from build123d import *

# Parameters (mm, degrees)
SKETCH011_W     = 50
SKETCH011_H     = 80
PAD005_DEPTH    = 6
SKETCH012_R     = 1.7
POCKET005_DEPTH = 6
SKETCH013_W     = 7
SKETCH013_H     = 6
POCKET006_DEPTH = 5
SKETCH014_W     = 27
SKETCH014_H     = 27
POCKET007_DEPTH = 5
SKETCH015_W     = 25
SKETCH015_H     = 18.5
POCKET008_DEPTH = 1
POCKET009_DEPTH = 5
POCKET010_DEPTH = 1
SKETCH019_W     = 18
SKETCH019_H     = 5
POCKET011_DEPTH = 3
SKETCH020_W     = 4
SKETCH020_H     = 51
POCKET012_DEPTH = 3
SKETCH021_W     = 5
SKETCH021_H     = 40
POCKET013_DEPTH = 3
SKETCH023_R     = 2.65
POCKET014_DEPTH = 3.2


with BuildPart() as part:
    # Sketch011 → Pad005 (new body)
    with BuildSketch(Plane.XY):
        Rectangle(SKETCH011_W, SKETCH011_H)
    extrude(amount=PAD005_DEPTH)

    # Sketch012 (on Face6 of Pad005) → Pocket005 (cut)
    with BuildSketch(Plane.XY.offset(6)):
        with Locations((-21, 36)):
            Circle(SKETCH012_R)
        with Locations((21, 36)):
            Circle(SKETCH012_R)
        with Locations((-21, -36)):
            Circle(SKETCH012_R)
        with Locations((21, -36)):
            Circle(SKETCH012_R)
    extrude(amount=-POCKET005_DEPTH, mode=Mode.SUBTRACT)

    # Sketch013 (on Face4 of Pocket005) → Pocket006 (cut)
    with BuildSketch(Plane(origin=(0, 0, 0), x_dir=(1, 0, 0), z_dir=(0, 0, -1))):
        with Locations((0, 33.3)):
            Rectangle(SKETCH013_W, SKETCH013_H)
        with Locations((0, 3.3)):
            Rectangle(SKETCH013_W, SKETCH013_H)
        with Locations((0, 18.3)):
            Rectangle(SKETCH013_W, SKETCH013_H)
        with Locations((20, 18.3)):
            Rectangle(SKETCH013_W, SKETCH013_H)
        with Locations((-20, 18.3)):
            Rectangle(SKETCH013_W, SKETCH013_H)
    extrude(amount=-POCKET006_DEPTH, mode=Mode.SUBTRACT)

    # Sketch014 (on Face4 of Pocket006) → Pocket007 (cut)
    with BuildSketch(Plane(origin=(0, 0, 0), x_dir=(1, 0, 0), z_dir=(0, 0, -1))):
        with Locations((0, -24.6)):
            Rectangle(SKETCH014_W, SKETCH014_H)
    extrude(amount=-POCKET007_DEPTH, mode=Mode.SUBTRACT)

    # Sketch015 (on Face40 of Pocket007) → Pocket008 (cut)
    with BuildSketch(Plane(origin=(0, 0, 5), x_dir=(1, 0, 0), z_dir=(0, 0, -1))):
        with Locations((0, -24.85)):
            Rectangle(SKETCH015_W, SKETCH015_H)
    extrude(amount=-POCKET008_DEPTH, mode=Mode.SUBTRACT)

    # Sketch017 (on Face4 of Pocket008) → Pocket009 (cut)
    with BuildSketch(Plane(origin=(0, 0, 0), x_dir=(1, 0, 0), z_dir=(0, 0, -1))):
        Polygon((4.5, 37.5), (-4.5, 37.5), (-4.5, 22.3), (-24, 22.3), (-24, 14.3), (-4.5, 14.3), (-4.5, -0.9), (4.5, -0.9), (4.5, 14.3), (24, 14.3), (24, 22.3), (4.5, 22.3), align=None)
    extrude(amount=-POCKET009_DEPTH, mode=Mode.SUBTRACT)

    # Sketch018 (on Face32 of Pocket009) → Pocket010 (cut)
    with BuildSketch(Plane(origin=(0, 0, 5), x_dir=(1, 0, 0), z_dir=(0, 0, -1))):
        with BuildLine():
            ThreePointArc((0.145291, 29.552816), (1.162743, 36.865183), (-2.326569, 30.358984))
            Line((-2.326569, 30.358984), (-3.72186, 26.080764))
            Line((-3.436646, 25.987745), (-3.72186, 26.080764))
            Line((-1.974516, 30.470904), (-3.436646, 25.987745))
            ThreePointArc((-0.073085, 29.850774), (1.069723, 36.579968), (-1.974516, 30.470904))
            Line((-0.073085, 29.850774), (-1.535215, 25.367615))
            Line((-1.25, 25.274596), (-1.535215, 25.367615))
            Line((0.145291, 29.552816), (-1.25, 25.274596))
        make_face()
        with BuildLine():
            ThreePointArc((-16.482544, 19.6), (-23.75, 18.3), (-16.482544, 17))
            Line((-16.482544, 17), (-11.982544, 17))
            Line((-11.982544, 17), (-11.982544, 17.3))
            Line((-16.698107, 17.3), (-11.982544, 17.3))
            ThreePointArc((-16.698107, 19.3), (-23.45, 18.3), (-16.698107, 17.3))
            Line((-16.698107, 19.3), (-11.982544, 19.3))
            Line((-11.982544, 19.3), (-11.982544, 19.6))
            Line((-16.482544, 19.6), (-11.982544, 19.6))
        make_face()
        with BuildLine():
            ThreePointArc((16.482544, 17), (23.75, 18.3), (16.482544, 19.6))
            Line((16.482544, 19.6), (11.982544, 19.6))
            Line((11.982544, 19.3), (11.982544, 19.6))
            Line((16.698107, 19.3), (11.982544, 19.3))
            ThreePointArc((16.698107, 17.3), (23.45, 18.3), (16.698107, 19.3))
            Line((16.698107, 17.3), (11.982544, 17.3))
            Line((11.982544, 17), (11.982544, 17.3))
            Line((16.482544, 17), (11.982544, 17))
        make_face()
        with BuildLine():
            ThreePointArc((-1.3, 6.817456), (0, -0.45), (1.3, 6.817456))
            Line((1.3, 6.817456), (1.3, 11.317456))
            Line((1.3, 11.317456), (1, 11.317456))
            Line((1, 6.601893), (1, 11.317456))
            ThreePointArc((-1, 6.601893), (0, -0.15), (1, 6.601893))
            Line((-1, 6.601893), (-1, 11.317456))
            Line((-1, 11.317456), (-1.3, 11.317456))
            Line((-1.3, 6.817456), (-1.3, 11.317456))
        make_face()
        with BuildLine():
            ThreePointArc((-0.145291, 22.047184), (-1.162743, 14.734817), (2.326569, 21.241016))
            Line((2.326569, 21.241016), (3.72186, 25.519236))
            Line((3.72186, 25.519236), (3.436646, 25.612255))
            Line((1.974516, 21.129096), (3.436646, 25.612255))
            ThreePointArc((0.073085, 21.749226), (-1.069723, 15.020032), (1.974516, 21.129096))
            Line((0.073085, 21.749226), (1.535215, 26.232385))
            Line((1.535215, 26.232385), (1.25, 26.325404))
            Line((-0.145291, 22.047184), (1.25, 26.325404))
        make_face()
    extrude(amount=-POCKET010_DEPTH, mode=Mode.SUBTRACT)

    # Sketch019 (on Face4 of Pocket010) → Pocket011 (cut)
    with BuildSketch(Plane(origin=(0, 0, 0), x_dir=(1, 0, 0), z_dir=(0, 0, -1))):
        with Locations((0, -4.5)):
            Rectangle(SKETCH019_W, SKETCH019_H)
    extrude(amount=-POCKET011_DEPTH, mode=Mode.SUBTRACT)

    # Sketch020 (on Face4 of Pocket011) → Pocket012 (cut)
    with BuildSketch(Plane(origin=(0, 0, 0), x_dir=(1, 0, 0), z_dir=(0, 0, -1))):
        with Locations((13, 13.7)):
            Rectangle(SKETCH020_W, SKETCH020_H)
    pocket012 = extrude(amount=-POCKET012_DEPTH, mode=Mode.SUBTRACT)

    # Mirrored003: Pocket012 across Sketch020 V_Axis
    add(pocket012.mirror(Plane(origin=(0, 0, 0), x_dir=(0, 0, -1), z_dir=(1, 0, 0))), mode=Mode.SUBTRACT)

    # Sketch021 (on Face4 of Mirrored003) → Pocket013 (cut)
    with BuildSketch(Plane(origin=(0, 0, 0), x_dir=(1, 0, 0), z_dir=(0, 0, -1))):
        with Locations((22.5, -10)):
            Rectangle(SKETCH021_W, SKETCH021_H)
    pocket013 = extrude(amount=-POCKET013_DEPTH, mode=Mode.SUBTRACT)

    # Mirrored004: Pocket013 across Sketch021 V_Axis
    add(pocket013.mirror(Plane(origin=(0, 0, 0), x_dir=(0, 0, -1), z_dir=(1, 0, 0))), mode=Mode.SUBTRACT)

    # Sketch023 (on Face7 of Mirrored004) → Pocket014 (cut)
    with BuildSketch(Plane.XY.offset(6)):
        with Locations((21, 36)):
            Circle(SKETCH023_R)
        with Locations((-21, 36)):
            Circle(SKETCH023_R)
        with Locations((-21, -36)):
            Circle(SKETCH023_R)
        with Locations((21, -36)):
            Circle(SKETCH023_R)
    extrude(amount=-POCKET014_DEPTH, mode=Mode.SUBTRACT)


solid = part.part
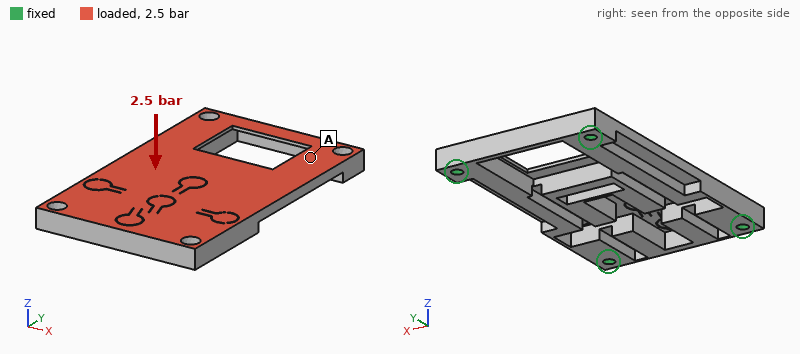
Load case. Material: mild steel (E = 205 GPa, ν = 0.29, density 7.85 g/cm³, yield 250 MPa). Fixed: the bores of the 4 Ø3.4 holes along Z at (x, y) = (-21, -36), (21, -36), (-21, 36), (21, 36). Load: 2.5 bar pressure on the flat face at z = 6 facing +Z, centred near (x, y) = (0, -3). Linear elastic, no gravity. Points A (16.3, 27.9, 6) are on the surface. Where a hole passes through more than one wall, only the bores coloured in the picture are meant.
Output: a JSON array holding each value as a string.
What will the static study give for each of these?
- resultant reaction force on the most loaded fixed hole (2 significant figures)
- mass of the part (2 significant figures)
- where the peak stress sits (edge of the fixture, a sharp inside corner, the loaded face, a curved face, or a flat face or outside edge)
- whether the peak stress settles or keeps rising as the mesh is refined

["370 N", "110 g", "a sharp inside corner", "keeps rising"]
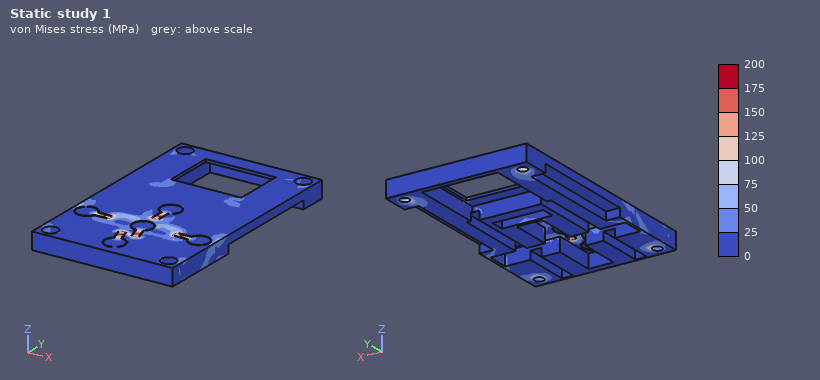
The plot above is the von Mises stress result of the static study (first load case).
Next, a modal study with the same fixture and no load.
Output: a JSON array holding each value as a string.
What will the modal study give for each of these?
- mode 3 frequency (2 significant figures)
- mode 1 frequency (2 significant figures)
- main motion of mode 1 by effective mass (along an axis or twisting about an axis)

["3300 Hz", "3100 Hz", "along Z"]
